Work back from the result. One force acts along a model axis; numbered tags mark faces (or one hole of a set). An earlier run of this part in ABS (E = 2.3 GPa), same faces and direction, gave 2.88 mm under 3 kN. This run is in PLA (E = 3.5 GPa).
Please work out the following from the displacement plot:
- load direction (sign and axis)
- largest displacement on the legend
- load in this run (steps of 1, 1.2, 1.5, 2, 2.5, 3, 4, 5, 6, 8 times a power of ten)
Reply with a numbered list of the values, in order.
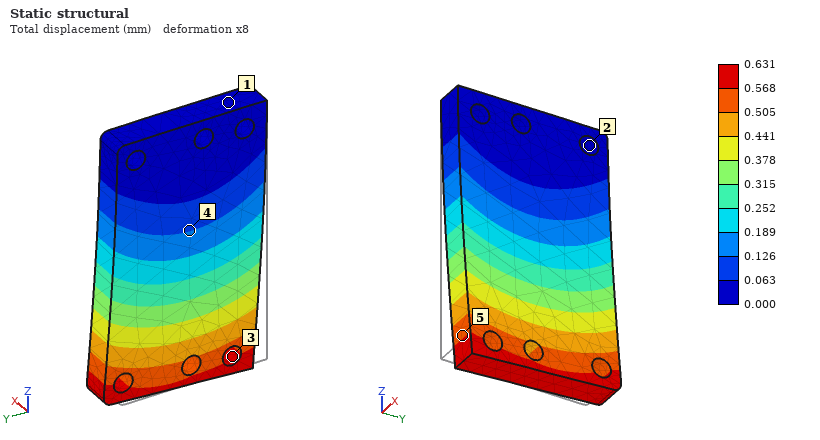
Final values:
1. +Y
2. 0.631 mm
3. 1 kN
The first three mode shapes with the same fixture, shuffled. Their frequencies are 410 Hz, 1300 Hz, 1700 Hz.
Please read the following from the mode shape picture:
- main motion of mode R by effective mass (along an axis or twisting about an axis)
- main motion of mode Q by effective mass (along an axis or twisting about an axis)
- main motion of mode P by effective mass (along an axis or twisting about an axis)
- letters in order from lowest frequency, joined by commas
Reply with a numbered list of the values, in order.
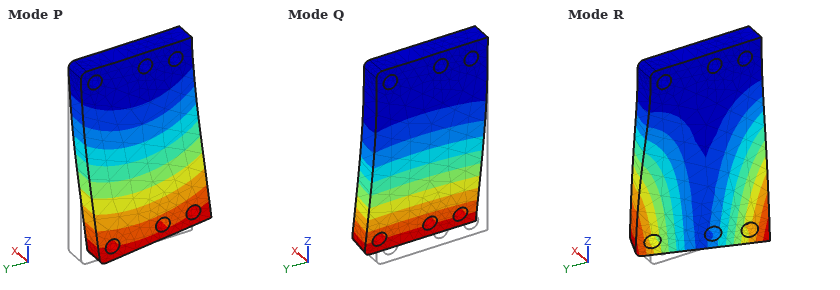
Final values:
1. twisting about Z
2. along X
3. along Y
4. Q, R, P
